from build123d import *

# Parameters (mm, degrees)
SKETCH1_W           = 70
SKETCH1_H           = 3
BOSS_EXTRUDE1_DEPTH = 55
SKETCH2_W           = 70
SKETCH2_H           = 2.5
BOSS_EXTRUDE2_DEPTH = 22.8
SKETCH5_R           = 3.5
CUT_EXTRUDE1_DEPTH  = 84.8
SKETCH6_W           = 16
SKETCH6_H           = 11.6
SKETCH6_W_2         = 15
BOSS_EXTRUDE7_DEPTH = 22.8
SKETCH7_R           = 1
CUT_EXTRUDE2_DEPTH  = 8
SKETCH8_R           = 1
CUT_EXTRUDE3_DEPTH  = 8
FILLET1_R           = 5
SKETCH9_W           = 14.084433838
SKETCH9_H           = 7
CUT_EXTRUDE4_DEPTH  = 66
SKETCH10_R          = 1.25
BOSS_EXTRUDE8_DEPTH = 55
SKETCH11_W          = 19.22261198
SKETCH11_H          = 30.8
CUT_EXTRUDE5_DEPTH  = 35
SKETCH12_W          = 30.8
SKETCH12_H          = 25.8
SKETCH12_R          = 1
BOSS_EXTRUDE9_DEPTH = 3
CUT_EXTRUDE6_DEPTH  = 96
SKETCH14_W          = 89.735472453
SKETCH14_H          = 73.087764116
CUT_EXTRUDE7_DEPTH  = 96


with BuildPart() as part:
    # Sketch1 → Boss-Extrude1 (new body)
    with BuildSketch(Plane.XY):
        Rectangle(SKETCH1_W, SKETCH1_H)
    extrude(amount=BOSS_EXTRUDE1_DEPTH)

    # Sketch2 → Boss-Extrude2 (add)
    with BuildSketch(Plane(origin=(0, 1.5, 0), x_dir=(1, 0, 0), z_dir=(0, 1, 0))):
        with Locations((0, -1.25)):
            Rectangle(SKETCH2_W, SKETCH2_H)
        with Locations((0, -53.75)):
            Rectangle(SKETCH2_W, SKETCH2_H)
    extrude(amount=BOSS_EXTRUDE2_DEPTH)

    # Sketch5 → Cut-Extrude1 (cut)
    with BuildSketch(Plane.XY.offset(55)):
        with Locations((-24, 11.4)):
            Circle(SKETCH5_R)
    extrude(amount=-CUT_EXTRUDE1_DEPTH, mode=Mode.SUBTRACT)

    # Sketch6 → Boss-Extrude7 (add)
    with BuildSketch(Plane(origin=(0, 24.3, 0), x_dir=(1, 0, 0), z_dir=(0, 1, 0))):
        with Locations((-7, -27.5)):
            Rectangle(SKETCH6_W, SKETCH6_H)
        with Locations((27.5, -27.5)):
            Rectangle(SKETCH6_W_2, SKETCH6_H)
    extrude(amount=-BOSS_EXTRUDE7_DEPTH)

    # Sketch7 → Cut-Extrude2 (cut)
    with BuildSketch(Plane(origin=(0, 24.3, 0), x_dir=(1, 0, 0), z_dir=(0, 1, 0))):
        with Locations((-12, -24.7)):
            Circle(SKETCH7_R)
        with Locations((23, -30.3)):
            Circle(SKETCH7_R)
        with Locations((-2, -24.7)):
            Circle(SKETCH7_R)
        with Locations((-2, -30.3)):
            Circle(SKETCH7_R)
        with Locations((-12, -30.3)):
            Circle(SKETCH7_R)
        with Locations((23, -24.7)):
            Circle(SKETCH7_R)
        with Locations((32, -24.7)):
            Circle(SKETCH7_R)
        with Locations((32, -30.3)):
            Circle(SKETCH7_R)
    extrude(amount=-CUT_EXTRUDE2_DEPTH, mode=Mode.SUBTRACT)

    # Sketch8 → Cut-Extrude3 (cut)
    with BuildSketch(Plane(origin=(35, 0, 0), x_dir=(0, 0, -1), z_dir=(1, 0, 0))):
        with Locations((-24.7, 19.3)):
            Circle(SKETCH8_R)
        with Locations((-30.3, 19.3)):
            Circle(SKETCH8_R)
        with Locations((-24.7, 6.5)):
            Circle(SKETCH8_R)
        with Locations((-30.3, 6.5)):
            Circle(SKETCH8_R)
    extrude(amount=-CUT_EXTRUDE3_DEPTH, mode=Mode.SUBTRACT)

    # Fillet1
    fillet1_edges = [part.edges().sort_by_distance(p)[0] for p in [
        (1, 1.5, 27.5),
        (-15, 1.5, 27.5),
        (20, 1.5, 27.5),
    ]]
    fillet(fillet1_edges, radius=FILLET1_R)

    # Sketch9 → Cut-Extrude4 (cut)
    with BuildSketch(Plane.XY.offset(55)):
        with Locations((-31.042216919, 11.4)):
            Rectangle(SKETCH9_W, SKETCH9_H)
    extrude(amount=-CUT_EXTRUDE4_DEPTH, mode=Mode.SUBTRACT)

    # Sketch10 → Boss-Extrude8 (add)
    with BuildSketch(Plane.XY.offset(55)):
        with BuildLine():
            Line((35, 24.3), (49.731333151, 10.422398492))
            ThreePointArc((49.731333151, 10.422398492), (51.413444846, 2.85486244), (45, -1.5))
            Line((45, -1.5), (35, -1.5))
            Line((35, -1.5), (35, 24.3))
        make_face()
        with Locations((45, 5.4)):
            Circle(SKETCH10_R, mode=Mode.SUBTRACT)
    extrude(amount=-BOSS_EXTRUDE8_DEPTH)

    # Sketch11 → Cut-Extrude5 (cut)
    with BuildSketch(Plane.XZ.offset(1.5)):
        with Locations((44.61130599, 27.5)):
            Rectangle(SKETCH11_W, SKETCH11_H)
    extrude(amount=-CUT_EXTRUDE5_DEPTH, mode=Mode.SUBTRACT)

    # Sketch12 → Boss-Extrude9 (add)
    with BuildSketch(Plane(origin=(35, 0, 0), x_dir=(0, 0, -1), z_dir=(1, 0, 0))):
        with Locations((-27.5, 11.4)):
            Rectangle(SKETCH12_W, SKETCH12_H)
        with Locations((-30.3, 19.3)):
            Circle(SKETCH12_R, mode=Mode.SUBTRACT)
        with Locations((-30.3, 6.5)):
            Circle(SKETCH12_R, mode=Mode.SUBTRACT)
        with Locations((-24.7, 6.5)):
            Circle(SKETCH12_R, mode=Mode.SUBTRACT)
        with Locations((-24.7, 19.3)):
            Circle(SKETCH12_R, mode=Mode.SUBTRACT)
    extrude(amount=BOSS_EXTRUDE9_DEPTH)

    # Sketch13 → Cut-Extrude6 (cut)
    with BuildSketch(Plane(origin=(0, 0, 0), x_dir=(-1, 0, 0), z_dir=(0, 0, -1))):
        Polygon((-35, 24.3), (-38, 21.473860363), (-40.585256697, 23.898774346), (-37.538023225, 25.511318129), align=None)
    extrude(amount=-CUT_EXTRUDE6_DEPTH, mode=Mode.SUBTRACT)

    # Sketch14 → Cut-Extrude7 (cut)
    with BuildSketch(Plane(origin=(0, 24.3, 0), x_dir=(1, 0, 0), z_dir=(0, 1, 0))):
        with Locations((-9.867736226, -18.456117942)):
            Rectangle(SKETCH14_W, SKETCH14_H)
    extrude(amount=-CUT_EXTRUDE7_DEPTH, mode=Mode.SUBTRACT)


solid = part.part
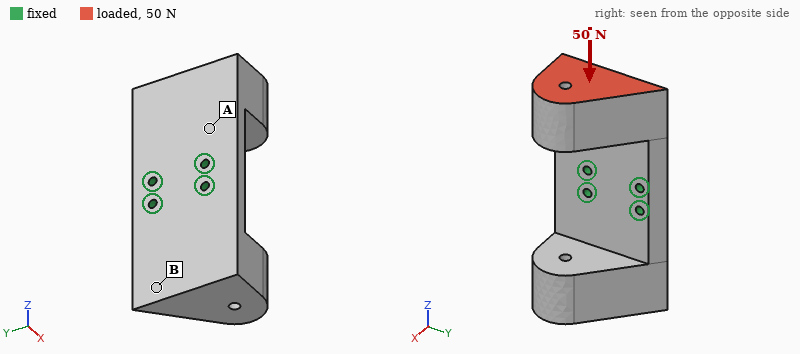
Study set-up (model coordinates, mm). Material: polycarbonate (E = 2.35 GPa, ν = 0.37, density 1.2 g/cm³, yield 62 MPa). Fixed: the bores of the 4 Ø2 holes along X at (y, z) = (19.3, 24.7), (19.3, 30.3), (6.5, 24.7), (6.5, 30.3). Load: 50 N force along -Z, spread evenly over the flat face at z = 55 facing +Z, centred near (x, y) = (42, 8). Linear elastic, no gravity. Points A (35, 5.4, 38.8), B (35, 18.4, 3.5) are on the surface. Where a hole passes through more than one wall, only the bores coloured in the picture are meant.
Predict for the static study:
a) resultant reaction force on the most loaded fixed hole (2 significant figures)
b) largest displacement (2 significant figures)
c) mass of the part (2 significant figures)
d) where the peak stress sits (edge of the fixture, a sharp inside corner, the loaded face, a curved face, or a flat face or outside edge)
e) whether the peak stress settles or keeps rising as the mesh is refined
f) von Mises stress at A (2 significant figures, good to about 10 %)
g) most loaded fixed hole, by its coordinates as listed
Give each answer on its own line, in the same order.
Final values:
30 N
0.67 mm
11 g
edge of the fixture
keeps rising
5.5 MPa
(6.5, 30.3)
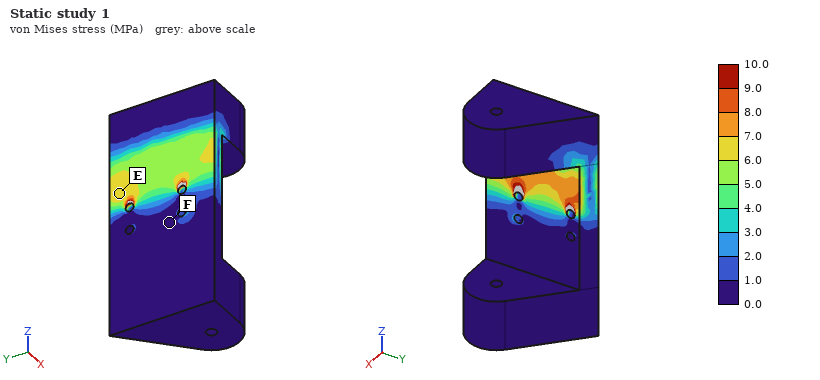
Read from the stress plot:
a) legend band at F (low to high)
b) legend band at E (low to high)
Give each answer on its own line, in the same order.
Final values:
0.0 to 1.0 MPa
6.0 to 7.0 MPa
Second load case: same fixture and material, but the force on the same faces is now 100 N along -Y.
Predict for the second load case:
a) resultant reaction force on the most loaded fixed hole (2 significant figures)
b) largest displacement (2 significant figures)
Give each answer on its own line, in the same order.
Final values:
140 N
0.39 mm
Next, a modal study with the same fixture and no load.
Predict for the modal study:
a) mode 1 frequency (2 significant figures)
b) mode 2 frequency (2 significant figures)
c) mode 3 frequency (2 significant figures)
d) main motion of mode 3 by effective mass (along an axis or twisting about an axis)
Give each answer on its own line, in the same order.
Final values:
510 Hz
510 Hz
1400 Hz
twisting about X
